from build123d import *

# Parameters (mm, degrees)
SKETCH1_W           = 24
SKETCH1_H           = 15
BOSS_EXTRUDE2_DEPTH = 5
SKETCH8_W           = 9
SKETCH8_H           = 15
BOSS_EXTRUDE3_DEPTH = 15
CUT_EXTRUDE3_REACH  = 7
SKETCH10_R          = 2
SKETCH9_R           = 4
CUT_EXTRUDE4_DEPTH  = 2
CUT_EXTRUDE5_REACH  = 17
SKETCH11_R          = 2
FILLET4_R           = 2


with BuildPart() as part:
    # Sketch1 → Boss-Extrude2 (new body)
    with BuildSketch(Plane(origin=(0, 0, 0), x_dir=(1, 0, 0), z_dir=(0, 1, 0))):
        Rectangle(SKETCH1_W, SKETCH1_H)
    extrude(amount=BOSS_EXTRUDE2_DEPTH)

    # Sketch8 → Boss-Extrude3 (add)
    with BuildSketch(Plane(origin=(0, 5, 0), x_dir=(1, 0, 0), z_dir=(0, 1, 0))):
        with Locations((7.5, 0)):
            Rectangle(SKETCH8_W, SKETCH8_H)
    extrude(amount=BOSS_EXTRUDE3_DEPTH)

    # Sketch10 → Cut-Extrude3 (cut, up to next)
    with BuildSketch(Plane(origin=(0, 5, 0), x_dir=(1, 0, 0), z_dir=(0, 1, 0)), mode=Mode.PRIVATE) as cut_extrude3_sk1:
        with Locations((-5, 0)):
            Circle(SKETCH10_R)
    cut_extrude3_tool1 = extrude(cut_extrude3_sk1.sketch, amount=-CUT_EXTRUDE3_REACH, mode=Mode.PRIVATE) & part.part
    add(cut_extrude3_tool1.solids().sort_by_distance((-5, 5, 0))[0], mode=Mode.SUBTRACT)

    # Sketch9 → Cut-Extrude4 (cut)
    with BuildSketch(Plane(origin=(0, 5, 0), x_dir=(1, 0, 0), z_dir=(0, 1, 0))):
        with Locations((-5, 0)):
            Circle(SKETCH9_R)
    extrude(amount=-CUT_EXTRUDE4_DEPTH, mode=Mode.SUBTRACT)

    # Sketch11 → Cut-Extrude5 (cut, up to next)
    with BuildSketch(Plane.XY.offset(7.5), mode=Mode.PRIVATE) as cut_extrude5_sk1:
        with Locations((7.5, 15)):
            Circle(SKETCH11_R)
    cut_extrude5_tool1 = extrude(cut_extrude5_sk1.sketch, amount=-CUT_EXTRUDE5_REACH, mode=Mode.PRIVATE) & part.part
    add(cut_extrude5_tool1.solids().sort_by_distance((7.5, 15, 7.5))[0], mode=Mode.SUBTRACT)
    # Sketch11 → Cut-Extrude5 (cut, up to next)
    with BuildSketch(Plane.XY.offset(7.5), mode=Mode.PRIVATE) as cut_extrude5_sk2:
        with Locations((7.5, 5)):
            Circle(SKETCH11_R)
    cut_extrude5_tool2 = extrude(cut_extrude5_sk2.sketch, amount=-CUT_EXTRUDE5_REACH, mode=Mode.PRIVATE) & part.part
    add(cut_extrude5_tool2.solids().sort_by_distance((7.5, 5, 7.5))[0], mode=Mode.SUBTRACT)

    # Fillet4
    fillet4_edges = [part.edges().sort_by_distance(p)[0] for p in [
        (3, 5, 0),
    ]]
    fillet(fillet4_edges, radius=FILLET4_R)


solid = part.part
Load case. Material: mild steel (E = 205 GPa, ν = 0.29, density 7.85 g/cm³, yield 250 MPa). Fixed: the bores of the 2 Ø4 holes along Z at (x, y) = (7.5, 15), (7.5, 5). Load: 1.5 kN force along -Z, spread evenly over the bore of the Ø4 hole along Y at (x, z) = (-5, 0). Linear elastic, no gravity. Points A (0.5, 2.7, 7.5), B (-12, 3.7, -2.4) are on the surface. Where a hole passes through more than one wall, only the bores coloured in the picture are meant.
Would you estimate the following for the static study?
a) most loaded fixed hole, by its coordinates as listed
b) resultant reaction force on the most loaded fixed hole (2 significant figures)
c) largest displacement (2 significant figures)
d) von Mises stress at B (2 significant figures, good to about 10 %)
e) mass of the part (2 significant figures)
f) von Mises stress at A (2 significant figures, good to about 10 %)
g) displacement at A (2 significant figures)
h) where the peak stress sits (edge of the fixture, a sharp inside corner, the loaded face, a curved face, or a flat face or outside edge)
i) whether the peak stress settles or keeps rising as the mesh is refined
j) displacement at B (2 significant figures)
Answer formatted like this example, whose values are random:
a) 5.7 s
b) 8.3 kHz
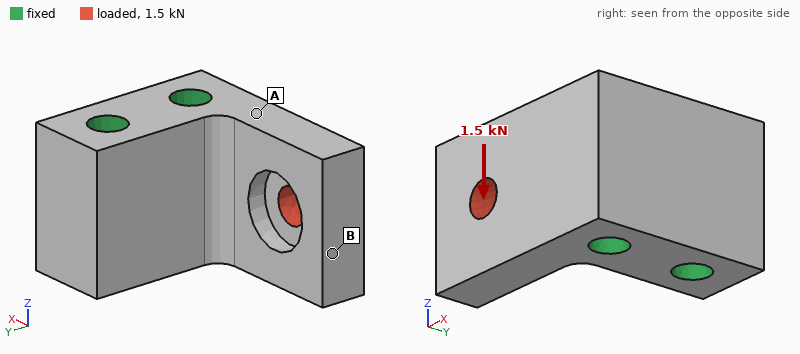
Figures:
a) (7.5, 5)
b) 1.5 kN
c) 10 µm
d) 14 MPa
e) 26 g
f) 54 MPa
g) 3.3 µm
h) edge of the fixture
i) keeps rising
j) 9.5 µm
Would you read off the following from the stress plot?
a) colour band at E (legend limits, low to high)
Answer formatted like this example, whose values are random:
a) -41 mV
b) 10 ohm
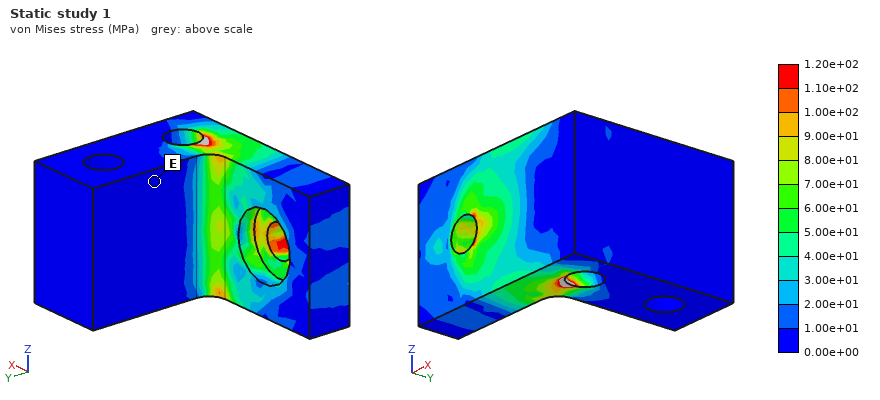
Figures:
a) 0.00e+00 to 1.00e+01 MPa
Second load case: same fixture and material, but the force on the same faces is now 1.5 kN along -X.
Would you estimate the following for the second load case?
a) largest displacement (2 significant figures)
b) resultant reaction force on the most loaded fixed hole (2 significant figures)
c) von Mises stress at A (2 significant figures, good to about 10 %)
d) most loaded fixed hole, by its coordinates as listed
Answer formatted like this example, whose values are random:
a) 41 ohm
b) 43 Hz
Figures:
a) 8.0 µm
b) 1.6 kN
c) 16 MPa
d) (7.5, 5)
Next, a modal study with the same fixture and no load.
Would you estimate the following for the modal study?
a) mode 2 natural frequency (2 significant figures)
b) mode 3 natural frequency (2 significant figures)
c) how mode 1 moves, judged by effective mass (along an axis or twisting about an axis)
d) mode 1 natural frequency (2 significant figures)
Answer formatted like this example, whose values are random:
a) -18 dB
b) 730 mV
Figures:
a) 24 kHz
b) 30 kHz
c) along Y
d) 14 kHz
